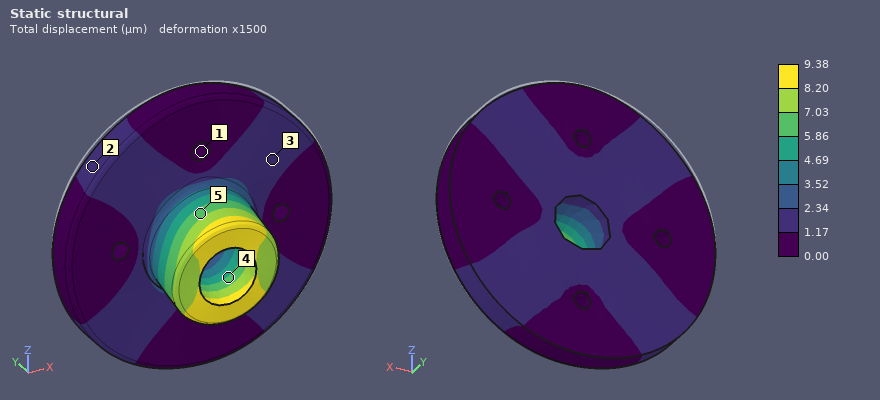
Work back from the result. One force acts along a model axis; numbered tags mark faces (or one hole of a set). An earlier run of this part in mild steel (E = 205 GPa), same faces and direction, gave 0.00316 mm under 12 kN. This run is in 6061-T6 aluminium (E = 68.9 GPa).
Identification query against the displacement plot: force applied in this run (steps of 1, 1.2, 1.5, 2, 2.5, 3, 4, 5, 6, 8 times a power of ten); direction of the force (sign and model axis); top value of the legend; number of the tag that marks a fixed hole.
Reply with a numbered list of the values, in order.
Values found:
1. 12 kN
2. -Z
3. 9.38 µm
4. 1
